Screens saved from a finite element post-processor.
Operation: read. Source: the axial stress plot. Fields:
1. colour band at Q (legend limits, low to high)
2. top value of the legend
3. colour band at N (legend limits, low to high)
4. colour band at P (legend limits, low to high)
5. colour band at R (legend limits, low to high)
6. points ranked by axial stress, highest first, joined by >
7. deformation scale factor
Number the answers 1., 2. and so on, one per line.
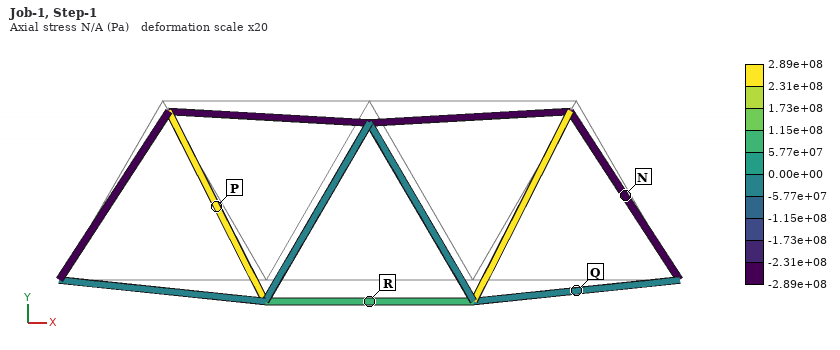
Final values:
1. -5.77e+07 to 0.00e+00 Pa
2. 2.89e+08 Pa
3. -2.89e+08 to -2.31e+08 Pa
4. 2.31e+08 to 2.89e+08 Pa
5. 5.77e+07 to 1.15e+08 Pa
6. P > R > Q > N
7. 20
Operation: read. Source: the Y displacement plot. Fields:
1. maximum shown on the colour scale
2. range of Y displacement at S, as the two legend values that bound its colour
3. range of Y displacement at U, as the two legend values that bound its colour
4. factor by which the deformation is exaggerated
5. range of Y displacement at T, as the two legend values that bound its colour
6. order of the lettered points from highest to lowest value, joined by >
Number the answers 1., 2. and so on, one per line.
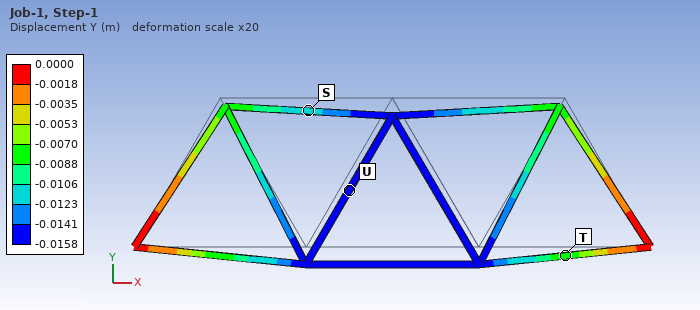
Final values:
1. 0.0000 m
2. -0.0123 to -0.0106 m
3. -0.0158 to -0.0141 m
4. 20
5. -0.0088 to -0.0070 m
6. T > S > U
